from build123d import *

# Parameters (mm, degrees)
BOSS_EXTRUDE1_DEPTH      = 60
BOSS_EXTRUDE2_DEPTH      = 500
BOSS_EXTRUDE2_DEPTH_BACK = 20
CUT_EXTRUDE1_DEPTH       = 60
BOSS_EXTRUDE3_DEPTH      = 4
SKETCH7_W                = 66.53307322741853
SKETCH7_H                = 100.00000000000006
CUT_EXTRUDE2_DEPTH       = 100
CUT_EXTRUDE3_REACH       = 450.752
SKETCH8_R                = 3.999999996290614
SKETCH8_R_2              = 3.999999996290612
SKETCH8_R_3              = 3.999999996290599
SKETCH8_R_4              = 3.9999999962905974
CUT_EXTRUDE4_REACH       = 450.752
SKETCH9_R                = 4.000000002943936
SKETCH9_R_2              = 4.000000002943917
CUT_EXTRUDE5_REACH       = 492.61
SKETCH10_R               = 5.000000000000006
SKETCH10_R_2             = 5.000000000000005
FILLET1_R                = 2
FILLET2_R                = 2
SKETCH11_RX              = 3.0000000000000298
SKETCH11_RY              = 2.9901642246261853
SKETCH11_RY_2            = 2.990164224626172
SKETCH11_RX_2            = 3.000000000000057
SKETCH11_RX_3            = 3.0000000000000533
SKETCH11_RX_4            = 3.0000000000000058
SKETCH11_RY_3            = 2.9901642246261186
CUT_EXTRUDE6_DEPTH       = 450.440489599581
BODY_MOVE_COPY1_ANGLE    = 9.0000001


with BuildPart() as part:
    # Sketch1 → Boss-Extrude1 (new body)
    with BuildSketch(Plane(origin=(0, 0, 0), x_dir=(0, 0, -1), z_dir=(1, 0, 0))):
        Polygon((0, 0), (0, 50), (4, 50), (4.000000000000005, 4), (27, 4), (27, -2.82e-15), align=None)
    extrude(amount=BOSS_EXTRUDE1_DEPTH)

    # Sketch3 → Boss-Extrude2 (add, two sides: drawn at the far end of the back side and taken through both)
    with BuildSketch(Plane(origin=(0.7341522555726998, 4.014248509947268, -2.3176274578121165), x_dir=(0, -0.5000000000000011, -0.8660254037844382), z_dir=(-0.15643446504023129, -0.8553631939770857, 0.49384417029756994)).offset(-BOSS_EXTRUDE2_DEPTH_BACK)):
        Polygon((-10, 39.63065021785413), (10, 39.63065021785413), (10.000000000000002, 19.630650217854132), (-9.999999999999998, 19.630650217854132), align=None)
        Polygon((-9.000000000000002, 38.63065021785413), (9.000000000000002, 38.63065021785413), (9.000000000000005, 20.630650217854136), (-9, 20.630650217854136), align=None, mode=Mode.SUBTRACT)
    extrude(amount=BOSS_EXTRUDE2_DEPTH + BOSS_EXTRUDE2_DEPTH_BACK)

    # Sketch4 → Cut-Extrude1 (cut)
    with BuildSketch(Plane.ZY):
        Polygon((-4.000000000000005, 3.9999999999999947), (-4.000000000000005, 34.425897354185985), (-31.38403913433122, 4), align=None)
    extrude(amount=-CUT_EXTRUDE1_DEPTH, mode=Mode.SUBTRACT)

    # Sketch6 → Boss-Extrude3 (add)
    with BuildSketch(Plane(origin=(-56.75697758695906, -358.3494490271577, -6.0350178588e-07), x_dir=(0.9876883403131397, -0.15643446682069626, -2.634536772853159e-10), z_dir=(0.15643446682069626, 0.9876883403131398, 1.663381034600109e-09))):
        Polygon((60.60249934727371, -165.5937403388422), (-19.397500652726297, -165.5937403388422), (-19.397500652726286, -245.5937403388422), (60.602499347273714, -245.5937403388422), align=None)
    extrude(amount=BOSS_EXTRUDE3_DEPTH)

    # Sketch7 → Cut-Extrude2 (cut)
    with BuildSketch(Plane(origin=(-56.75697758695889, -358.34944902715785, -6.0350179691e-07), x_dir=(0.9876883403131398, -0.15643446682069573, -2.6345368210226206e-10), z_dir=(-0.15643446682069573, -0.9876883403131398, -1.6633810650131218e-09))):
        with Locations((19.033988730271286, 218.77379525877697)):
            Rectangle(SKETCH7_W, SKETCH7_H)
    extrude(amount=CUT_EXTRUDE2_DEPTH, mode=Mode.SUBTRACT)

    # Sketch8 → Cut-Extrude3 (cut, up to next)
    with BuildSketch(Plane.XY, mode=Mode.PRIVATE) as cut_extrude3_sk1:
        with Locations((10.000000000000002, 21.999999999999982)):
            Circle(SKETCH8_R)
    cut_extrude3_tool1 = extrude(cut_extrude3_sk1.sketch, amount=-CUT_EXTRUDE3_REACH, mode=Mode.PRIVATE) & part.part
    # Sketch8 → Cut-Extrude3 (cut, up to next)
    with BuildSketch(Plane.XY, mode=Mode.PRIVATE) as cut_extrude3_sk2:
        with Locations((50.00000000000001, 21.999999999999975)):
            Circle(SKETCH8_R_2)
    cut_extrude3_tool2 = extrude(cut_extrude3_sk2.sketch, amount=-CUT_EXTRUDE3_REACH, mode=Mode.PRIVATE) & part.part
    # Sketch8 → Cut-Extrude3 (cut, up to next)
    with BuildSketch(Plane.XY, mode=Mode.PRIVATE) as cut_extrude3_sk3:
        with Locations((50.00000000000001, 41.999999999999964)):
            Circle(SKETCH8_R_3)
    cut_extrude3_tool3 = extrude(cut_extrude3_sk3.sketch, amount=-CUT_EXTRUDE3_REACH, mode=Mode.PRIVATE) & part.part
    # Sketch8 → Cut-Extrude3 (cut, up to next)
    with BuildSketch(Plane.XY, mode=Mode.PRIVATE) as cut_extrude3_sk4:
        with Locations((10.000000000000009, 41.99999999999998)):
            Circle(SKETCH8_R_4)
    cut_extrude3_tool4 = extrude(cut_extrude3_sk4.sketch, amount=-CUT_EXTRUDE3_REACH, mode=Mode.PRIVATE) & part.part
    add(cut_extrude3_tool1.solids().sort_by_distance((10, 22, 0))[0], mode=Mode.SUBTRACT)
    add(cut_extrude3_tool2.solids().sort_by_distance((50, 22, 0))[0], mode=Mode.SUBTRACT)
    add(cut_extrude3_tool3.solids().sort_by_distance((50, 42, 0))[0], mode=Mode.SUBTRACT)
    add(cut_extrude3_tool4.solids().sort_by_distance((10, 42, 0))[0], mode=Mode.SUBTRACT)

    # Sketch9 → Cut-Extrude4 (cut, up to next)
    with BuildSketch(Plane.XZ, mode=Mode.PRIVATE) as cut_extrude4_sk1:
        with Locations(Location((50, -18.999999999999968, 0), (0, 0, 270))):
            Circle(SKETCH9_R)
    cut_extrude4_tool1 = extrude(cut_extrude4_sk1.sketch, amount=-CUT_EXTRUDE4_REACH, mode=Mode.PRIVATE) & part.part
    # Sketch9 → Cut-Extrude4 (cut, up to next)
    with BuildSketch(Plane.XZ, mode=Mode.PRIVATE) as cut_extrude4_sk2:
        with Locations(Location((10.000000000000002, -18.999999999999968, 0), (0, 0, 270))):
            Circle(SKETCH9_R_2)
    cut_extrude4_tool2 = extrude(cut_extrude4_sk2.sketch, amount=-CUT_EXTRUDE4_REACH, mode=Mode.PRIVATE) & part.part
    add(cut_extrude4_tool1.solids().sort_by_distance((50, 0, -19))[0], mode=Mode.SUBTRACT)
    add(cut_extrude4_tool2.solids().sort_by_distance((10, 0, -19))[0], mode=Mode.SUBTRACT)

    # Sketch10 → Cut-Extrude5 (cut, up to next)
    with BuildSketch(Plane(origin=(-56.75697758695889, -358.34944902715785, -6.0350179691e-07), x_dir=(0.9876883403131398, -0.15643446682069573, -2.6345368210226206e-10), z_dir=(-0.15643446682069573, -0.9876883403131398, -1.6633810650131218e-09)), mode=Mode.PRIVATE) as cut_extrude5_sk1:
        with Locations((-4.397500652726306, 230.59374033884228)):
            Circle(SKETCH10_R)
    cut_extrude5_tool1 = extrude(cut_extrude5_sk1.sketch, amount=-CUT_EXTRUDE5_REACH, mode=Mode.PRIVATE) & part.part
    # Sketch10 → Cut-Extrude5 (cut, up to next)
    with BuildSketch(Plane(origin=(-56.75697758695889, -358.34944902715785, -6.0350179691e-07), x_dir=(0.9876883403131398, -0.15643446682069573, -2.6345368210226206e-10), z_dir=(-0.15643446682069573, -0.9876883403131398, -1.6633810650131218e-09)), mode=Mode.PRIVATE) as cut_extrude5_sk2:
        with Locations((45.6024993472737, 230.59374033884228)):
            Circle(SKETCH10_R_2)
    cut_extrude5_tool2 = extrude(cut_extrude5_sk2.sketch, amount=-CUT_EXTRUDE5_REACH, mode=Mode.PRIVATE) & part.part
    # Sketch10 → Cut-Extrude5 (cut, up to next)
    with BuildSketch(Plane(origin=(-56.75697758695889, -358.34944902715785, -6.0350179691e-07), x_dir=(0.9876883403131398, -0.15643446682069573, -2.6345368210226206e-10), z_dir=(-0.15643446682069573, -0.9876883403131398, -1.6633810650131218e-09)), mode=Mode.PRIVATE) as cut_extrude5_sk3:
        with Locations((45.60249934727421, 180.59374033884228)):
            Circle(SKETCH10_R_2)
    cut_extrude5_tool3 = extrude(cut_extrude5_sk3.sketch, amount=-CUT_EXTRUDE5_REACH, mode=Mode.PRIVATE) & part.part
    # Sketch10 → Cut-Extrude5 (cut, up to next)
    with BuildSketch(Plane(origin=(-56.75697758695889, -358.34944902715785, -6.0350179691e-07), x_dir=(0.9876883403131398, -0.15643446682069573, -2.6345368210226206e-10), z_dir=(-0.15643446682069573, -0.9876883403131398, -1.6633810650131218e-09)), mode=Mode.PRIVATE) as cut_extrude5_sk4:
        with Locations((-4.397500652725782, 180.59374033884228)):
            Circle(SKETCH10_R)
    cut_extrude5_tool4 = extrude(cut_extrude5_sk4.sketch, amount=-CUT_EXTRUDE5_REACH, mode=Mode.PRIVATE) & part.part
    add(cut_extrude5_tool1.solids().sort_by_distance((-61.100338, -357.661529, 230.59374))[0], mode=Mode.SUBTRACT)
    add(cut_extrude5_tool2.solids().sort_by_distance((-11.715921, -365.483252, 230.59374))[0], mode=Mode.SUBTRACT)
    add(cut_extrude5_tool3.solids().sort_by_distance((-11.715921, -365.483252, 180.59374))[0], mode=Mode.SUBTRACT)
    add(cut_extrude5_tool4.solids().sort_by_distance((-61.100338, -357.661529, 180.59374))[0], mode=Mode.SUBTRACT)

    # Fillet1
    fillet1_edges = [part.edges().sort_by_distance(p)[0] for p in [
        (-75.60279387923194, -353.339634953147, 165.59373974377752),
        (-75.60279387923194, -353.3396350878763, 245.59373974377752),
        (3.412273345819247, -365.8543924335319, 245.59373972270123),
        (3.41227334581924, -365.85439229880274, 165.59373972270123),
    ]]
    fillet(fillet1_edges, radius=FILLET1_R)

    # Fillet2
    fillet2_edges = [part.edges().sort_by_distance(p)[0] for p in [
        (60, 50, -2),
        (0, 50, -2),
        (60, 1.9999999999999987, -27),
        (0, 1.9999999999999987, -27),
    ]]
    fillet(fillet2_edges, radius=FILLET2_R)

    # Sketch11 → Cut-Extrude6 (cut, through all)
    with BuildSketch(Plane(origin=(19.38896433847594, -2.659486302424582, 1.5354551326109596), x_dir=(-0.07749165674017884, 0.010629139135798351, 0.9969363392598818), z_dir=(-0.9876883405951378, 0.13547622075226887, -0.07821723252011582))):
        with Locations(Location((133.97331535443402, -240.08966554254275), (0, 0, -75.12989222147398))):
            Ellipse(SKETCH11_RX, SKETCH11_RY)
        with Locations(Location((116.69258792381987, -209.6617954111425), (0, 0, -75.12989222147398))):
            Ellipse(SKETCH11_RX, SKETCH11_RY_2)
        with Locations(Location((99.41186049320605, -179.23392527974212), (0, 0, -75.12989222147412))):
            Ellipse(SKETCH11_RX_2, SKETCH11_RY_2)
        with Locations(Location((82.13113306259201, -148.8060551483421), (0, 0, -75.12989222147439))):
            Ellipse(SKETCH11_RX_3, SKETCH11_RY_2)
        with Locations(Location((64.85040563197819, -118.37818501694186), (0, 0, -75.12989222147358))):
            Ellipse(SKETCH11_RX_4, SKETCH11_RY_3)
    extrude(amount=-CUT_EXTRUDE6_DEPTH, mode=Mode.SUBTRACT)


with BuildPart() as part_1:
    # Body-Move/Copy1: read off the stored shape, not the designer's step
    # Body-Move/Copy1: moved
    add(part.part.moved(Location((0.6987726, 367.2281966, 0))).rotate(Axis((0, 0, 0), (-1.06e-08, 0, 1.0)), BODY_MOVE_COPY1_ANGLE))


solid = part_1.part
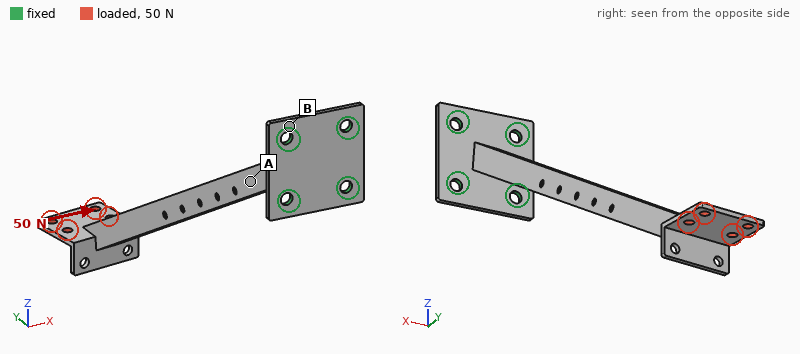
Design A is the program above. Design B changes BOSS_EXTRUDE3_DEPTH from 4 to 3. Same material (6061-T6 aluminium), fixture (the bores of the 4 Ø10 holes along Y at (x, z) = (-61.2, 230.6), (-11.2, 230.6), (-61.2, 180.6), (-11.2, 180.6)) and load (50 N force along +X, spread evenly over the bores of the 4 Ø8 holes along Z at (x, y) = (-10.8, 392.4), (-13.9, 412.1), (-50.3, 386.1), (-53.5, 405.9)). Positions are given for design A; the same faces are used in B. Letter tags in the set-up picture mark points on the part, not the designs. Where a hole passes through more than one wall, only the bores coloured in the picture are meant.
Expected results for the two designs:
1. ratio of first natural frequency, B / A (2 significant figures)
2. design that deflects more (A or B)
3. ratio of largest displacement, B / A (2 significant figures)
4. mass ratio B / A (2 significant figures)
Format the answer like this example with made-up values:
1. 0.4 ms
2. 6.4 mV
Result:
1. 0.92
2. B
3. 1.1
4. 0.92
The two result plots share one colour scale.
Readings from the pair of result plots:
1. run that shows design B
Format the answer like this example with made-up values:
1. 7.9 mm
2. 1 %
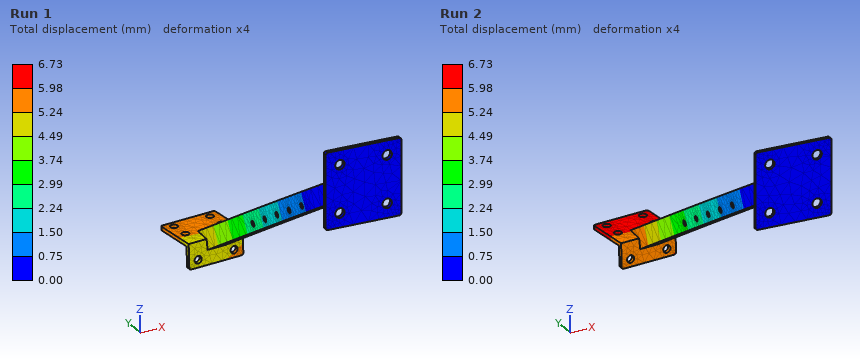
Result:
1. Run 2
